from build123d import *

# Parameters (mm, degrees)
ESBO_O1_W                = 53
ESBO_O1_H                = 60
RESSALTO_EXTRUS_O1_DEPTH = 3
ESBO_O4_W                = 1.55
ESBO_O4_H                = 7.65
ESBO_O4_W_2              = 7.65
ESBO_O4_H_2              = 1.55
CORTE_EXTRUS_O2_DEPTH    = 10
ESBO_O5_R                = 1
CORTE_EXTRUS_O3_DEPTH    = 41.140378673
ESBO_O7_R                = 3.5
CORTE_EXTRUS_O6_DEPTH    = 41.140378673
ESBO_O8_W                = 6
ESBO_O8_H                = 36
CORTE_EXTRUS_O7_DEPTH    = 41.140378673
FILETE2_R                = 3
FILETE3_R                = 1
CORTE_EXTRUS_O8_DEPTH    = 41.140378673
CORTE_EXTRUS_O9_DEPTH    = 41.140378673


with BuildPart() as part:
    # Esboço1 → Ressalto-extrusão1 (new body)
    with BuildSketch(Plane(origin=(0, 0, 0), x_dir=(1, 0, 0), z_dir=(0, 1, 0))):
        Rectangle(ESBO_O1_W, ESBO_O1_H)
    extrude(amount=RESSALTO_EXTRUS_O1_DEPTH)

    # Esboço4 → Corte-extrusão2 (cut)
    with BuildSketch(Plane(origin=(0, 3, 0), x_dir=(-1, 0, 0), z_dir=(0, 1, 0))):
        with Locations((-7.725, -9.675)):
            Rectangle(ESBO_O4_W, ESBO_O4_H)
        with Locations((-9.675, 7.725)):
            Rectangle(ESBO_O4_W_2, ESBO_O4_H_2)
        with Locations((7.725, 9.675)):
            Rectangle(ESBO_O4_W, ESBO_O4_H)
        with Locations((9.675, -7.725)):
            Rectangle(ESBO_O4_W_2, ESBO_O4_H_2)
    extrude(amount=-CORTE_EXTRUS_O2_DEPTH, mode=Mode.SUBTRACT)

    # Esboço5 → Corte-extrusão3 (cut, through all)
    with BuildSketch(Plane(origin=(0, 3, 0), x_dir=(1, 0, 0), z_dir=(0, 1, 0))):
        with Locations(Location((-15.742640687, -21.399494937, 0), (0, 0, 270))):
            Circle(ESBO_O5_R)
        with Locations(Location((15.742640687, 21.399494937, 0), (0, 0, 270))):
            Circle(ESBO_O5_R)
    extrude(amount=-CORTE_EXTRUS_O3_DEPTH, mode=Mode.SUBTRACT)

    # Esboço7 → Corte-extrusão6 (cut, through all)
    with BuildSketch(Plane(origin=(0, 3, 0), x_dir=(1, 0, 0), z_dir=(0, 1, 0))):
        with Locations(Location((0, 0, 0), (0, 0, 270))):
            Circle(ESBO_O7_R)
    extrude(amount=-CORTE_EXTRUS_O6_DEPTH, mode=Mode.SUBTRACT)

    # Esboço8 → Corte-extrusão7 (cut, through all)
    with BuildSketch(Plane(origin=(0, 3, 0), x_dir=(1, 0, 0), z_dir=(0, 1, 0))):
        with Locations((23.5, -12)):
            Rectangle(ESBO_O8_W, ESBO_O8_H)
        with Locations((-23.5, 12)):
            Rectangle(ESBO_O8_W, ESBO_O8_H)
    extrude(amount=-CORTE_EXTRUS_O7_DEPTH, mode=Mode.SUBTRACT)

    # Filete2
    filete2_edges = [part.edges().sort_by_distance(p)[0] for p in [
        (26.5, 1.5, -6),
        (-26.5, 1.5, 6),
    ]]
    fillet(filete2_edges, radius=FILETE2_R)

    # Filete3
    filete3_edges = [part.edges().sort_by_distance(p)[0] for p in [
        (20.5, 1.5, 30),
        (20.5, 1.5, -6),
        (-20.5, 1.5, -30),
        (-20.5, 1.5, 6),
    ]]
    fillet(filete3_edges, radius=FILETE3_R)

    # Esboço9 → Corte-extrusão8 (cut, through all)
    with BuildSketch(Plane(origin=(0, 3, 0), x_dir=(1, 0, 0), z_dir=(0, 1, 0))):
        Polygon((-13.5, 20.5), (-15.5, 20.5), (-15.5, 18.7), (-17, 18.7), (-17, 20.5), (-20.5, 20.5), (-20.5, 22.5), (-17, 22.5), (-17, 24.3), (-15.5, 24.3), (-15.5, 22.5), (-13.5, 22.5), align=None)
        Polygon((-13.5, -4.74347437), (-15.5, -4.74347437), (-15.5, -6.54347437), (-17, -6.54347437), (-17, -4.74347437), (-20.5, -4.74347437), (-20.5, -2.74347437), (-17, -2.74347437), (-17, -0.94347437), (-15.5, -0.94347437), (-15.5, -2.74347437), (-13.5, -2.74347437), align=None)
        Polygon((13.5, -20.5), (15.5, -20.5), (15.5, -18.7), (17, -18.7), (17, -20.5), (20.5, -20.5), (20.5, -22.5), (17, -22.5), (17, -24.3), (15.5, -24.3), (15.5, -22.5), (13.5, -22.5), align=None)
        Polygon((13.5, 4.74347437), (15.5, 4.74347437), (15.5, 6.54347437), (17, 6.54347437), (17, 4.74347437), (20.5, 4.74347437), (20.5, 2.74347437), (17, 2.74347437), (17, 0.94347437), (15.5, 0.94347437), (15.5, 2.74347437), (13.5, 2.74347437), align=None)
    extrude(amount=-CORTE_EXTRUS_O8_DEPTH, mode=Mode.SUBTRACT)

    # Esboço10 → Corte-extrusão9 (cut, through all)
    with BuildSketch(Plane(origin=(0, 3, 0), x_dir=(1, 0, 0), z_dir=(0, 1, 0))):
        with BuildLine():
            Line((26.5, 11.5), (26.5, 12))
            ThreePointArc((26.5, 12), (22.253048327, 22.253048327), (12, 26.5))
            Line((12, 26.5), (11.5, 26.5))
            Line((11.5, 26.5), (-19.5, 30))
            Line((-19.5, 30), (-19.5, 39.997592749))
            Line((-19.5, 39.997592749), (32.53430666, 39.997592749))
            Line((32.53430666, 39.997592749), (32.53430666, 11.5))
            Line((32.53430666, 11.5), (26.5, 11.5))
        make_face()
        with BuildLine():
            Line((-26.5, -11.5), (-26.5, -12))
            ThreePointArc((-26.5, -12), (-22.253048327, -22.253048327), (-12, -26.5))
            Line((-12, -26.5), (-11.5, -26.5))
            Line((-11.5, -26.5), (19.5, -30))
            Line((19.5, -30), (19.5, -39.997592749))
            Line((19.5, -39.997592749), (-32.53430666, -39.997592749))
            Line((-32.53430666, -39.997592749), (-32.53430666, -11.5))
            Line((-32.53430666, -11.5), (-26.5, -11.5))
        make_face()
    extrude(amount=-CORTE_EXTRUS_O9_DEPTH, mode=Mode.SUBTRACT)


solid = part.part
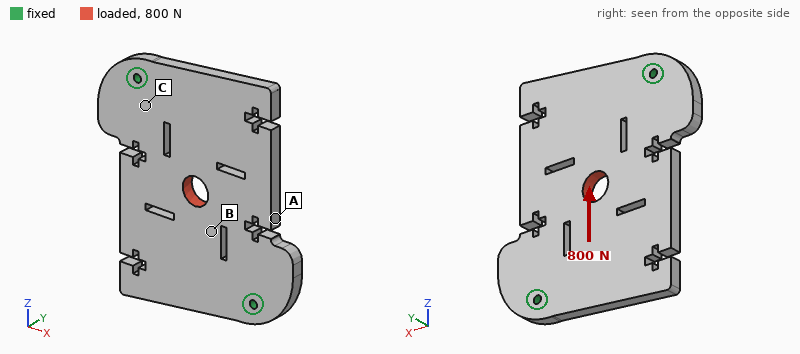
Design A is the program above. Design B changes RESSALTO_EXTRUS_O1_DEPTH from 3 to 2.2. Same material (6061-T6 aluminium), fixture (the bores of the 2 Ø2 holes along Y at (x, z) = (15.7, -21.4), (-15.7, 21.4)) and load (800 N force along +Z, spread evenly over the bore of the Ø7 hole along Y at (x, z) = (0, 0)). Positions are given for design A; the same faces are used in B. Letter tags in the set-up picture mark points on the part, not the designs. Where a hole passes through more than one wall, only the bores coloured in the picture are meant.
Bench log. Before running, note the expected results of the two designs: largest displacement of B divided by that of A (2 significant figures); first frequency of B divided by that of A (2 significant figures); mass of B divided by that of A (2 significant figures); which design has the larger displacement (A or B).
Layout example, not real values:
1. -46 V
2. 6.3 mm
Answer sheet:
1. 1.4
2. 0.75
3. 0.73
4. B
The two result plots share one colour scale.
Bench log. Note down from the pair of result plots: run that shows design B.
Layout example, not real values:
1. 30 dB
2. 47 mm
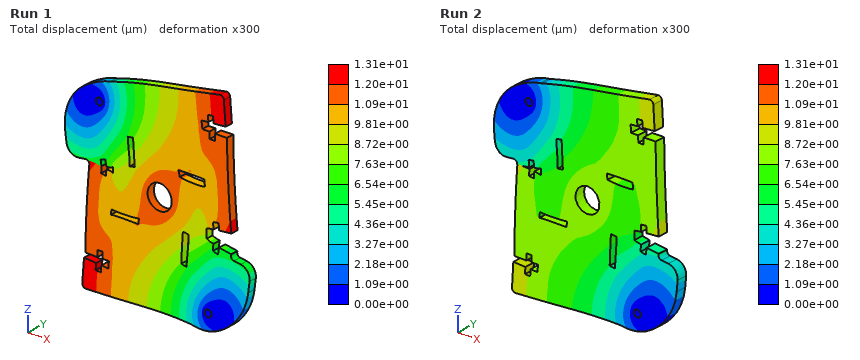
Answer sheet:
1. Run 1
